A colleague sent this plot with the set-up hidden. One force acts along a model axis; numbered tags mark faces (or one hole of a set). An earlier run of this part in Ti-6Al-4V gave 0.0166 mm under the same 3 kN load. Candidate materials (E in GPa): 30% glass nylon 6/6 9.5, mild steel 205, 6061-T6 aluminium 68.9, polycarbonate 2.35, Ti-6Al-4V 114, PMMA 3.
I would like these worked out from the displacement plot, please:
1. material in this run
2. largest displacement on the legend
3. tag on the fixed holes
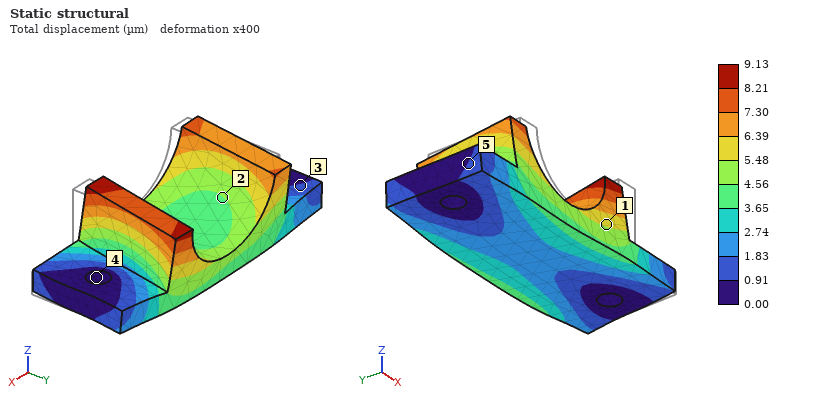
mild steel
9.13 µm
4
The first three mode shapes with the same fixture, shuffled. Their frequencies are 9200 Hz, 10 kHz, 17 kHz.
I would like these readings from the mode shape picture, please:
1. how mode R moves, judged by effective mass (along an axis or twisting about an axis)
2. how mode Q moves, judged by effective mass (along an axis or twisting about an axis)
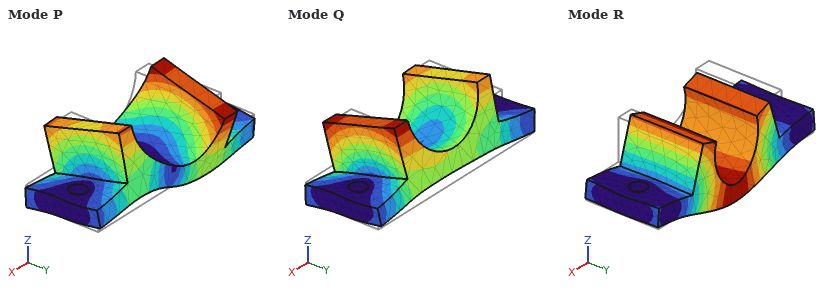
along Z
along Y
